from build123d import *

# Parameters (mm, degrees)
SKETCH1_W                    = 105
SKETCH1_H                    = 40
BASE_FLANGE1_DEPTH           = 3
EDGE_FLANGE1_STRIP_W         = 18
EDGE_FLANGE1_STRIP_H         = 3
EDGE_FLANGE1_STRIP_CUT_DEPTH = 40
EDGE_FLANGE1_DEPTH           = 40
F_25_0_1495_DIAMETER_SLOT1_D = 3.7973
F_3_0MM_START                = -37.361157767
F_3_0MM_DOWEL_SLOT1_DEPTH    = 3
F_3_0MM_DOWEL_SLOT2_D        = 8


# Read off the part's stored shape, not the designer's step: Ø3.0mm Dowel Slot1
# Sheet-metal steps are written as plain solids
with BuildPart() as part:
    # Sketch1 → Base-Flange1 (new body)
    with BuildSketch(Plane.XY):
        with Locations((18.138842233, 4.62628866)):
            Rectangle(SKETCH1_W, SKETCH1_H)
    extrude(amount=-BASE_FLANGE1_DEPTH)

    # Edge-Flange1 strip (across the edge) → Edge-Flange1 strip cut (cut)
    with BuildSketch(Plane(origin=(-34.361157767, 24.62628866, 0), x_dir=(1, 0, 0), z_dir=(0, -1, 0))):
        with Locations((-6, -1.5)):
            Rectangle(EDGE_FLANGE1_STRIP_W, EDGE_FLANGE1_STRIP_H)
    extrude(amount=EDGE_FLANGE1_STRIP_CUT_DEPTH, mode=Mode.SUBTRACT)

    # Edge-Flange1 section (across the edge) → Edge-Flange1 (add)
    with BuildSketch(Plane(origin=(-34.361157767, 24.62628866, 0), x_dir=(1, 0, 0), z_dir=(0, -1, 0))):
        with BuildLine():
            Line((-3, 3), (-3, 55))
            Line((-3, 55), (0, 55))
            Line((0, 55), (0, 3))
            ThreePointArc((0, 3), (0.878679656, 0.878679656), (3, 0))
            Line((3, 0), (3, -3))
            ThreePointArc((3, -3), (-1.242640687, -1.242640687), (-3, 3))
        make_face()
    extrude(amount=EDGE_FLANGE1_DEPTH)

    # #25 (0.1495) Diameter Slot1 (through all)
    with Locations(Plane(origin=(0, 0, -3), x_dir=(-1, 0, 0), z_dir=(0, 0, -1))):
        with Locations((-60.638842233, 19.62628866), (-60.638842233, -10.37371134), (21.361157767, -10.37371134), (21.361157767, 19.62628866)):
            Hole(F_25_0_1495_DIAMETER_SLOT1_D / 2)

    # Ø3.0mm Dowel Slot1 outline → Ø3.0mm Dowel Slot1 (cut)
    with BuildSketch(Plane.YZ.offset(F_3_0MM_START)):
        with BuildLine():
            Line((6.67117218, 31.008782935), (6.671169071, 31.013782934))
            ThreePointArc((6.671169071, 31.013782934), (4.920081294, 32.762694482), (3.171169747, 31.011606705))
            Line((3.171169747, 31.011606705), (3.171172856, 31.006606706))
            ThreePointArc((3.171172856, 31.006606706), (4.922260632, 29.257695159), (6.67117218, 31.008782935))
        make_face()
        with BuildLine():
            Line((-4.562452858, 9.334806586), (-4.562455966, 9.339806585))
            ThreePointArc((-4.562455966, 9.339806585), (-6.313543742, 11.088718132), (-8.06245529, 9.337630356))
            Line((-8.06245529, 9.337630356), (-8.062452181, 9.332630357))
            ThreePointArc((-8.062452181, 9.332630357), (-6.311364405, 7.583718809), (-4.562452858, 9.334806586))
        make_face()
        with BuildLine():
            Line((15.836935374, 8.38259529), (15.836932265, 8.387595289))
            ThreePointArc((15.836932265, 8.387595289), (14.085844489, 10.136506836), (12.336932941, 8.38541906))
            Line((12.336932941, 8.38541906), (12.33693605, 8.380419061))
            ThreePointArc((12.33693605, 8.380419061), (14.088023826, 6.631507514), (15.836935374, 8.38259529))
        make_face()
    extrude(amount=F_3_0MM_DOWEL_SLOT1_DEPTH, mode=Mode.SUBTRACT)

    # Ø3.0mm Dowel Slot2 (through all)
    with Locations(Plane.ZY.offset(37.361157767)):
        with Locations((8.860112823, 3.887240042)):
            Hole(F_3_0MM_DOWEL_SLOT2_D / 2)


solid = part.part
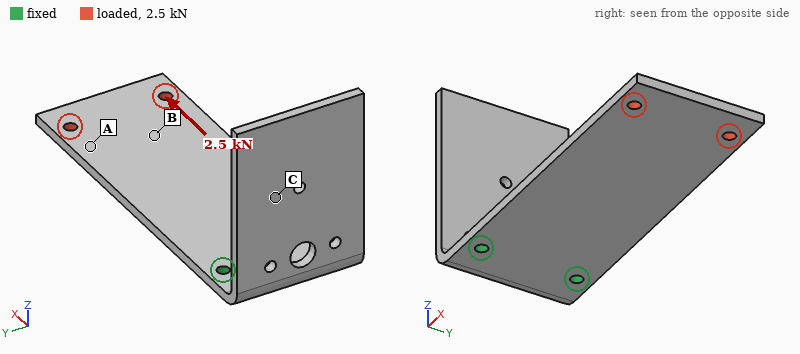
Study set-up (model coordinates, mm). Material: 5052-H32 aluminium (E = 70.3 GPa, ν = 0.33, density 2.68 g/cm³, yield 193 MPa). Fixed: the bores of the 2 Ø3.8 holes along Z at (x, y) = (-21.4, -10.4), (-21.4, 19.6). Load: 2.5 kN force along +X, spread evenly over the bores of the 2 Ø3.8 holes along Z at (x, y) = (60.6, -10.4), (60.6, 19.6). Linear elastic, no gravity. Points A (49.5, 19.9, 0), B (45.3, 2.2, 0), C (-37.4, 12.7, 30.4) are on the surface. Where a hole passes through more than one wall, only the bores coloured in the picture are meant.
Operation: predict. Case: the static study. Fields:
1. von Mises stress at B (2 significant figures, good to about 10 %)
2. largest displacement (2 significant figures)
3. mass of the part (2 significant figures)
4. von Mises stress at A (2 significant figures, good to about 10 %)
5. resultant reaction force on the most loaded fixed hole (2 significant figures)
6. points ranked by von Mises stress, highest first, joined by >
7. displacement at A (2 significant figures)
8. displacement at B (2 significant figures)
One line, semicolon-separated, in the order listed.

15 MPa; 30 µm; 51 g; 26 MPa; 1.3 kN; A > B > C; 23 µm; 21 µm
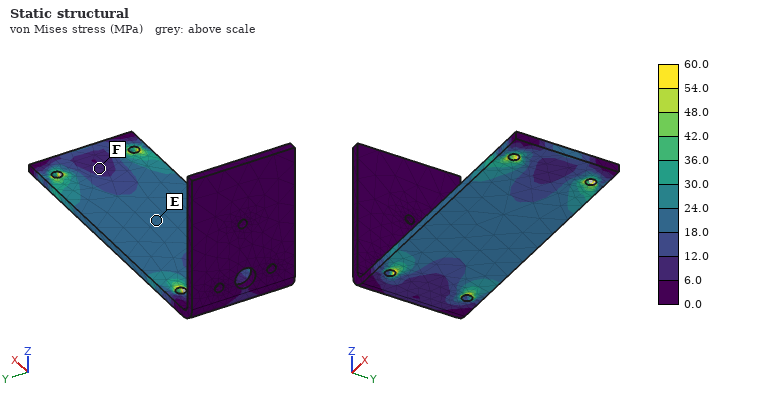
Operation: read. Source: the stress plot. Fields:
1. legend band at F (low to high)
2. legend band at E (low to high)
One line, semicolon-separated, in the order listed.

6.0 to 12.0 MPa; 18.0 to 24.0 MPa
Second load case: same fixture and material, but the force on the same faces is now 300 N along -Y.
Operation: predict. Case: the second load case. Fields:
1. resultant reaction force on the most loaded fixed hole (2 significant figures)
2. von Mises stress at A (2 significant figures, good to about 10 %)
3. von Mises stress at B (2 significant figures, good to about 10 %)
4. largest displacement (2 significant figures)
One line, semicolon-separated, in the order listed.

810 N; 4.1 MPa; 6.4 MPa; 71 µm
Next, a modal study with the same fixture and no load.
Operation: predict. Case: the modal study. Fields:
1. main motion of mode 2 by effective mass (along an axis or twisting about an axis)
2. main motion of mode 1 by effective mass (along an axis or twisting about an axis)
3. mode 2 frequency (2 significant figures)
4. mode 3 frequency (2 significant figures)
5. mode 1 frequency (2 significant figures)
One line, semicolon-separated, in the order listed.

along X; along Z; 550 Hz; 1400 Hz; 290 Hz
